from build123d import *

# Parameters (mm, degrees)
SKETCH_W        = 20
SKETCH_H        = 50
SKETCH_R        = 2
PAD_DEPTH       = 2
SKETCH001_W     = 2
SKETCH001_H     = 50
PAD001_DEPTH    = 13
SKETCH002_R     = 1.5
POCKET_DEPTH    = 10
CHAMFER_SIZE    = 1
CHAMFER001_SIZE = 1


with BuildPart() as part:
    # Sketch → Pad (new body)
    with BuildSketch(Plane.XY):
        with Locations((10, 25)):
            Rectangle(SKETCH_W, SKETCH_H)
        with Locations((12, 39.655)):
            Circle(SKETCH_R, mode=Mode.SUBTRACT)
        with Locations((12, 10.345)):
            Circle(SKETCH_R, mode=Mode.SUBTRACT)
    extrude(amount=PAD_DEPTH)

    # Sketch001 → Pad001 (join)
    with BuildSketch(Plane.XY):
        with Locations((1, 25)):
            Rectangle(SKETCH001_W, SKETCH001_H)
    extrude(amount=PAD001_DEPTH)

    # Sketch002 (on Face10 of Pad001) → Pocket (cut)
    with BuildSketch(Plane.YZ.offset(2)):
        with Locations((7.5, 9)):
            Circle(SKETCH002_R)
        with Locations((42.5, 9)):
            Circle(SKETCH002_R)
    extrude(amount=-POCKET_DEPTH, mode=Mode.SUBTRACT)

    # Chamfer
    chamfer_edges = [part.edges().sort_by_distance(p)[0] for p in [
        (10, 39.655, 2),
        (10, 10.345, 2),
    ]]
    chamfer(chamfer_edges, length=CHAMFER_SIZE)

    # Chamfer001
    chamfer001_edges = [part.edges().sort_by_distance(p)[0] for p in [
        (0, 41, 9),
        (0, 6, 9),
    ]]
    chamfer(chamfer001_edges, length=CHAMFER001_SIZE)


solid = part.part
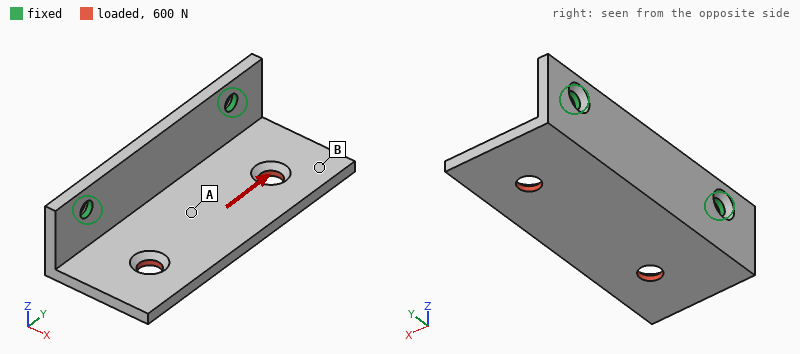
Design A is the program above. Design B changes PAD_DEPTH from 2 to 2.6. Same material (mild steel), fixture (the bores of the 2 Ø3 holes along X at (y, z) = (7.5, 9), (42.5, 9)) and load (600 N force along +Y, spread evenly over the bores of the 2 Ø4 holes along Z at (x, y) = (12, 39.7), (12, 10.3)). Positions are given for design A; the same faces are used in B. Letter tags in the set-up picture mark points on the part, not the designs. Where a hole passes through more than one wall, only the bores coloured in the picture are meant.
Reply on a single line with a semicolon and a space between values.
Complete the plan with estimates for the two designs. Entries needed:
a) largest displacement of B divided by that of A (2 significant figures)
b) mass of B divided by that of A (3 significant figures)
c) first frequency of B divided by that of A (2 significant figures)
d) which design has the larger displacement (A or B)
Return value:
0.72; 1.18; 0.94; A
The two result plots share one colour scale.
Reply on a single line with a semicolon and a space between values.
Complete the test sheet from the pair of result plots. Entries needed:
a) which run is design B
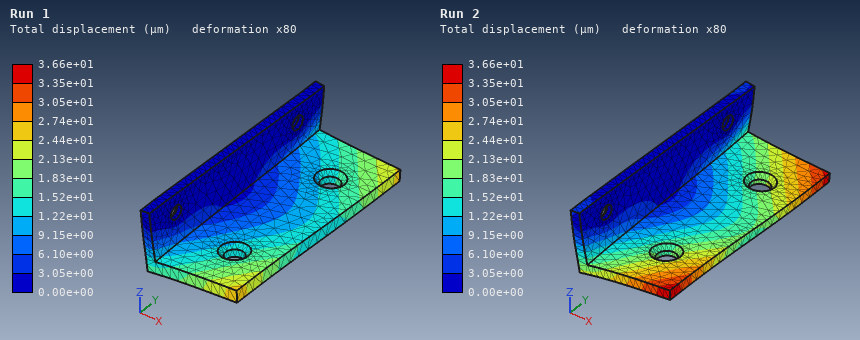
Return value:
Run 1
